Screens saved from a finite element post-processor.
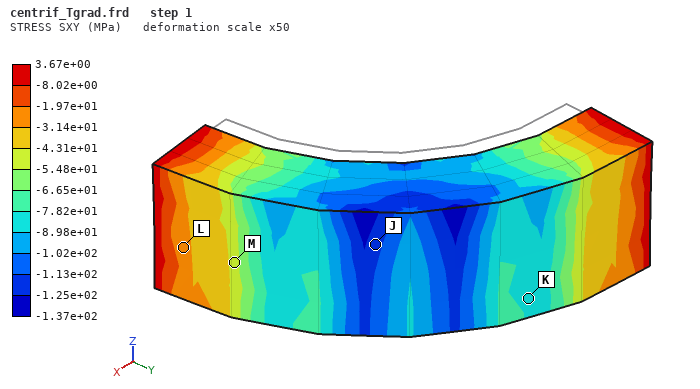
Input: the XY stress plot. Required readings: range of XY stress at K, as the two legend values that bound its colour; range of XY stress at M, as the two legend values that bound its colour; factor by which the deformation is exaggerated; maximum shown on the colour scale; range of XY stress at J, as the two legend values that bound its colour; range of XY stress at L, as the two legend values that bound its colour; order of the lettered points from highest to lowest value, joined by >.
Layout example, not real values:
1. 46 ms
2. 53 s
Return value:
1. -8.98e+01 to -7.82e+01 MPa
2. -5.48e+01 to -4.31e+01 MPa
3. 50
4. 3.67e+00 MPa
5. -1.25e+02 to -1.13e+02 MPa
6. -3.14e+01 to -1.97e+01 MPa
7. L > M > K > J
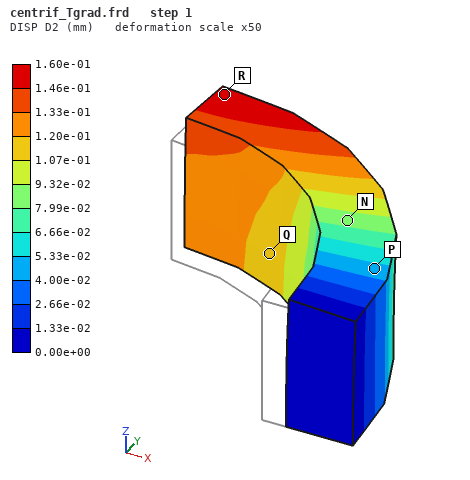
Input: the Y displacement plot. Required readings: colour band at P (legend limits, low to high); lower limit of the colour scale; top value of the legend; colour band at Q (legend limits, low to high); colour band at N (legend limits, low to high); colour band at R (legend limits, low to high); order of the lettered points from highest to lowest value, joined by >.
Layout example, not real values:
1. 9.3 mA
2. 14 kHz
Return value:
1. 4.00e-02 to 5.33e-02 mm
2. 0.00e+00 mm
3. 1.60e-01 mm
4. 1.07e-01 to 1.20e-01 mm
5. 7.99e-02 to 9.32e-02 mm
6. 1.46e-01 to 1.60e-01 mm
7. R > Q > N > P
